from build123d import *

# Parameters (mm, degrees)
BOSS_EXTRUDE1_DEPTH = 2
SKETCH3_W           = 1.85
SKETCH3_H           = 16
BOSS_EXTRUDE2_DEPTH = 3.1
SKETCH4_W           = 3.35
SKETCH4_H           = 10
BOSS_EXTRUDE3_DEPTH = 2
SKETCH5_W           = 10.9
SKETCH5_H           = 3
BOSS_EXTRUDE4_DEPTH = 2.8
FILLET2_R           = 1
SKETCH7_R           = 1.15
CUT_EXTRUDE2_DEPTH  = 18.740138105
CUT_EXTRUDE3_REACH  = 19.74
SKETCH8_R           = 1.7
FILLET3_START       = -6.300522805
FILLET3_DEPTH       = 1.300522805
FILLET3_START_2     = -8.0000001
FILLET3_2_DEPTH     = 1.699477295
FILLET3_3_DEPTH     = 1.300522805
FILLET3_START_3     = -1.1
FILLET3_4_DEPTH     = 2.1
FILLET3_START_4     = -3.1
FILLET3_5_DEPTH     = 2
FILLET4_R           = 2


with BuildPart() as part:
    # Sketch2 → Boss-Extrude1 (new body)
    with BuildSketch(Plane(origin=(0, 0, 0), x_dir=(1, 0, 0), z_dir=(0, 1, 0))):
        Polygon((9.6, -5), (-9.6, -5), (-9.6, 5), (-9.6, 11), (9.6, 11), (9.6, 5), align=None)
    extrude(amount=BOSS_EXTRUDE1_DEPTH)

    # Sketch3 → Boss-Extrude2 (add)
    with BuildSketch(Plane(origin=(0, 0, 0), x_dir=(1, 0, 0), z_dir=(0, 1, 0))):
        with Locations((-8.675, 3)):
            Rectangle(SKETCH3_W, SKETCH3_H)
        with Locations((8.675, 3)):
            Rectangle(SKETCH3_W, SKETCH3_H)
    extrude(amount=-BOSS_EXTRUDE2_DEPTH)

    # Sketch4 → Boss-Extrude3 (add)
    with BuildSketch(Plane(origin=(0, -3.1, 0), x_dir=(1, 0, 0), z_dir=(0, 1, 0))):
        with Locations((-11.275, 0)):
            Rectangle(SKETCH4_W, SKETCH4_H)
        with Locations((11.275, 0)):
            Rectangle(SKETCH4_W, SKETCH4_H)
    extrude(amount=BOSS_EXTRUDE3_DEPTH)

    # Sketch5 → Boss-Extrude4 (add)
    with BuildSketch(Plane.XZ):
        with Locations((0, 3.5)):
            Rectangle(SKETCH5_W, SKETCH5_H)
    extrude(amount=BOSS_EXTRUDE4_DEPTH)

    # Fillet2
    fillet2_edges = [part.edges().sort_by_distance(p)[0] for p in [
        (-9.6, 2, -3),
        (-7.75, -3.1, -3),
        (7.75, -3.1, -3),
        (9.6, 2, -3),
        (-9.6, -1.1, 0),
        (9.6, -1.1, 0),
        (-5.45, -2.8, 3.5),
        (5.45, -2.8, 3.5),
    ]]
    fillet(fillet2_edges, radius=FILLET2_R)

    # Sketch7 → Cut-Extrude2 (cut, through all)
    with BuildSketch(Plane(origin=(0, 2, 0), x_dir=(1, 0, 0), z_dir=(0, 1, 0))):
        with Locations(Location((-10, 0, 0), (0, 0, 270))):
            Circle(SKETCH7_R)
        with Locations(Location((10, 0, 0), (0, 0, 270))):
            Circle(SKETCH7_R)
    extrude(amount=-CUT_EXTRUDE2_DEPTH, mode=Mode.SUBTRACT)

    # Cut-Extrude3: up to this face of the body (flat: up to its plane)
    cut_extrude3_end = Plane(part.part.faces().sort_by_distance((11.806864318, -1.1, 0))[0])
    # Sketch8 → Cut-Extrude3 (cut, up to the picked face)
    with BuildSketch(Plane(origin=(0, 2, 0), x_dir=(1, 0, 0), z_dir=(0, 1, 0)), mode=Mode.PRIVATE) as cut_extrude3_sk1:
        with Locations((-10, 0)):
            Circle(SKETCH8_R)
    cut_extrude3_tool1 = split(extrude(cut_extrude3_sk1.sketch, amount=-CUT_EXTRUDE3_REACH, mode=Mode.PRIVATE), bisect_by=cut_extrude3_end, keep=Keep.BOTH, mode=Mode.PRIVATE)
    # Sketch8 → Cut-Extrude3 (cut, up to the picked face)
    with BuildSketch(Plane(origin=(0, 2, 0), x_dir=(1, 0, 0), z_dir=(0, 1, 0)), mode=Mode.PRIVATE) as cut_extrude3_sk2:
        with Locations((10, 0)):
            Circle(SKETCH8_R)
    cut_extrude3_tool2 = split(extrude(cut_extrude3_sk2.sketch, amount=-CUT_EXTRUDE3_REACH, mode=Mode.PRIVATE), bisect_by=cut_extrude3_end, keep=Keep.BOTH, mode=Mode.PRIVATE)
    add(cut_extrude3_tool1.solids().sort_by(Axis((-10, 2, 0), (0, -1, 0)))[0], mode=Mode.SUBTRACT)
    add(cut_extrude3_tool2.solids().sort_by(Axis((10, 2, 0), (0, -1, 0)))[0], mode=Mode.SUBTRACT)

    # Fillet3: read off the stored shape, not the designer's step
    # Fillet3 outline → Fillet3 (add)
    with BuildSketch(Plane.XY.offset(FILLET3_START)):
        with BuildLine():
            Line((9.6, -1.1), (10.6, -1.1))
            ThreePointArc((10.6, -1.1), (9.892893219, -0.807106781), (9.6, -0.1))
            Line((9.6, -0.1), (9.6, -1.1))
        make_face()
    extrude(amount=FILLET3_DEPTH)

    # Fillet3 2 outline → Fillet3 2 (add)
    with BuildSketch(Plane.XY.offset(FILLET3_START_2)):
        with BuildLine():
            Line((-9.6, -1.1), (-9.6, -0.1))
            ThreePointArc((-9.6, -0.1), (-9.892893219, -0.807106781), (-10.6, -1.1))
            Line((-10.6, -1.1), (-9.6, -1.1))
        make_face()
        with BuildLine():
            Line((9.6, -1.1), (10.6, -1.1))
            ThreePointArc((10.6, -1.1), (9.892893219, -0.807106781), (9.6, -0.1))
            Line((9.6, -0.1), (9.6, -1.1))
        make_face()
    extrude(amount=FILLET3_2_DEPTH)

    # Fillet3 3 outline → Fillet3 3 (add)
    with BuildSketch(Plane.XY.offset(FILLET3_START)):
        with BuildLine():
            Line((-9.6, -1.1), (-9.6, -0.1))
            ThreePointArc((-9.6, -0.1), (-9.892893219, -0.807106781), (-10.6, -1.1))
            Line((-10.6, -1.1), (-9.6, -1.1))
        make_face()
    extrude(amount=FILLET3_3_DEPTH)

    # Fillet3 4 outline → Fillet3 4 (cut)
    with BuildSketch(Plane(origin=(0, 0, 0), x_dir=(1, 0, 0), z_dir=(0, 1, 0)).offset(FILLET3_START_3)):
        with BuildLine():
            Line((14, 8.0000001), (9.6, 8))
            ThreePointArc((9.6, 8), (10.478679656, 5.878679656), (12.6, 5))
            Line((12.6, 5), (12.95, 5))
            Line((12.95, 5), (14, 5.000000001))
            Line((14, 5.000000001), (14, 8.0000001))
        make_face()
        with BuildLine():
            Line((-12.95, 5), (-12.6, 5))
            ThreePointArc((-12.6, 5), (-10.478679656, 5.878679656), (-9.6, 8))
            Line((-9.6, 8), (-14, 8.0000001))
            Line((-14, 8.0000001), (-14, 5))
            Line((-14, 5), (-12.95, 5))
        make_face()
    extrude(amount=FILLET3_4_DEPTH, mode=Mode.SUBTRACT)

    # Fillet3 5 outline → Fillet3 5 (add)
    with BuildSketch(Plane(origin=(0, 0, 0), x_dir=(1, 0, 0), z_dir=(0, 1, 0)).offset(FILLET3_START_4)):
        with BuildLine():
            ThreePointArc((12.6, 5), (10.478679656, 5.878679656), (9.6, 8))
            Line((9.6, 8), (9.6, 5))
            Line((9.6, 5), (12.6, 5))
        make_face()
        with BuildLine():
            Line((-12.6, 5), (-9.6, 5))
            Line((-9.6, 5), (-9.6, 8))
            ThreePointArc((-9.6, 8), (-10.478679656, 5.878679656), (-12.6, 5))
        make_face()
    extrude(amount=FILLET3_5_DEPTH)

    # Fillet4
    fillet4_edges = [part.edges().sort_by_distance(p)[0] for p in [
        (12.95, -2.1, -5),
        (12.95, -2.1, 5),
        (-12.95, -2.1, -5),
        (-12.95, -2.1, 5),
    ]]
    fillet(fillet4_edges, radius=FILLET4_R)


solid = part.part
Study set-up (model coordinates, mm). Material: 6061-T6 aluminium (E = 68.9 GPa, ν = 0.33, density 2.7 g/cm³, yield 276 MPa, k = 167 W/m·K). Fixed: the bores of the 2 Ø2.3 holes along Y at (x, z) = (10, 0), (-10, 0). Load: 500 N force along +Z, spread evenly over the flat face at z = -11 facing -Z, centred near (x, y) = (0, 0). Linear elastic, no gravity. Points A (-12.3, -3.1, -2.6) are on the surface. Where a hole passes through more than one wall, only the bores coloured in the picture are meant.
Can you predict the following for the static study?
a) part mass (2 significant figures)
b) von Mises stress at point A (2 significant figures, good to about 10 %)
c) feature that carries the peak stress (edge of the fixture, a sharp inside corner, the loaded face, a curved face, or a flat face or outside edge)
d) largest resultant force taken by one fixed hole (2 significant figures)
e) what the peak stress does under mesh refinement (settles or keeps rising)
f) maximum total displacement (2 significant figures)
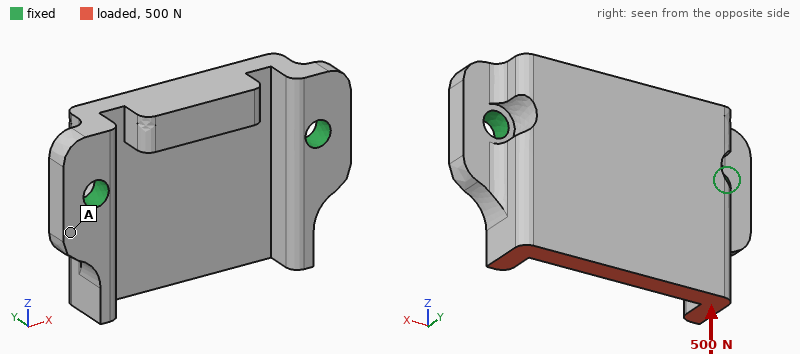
2.6 g
23 MPa
edge of the fixture
250 N
keeps rising
26 µm
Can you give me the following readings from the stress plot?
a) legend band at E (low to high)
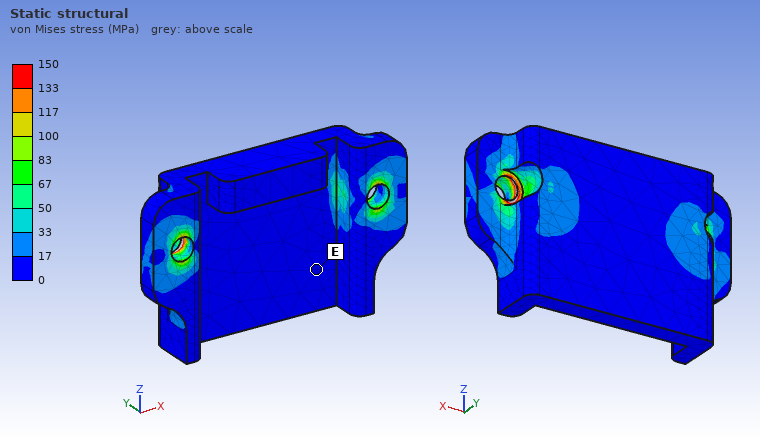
0 to 17 MPa
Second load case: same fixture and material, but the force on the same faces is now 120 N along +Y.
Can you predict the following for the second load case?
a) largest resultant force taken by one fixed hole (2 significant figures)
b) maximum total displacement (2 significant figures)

79 N
38 µm
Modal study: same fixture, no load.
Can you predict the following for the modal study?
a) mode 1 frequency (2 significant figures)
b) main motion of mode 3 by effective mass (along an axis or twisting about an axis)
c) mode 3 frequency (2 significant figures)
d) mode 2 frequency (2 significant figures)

13 kHz
along Y
26 kHz
22 kHz
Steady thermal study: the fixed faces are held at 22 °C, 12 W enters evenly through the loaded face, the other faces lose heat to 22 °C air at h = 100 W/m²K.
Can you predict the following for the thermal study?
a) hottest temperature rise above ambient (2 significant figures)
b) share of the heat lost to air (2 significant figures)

20 K
7.8 %
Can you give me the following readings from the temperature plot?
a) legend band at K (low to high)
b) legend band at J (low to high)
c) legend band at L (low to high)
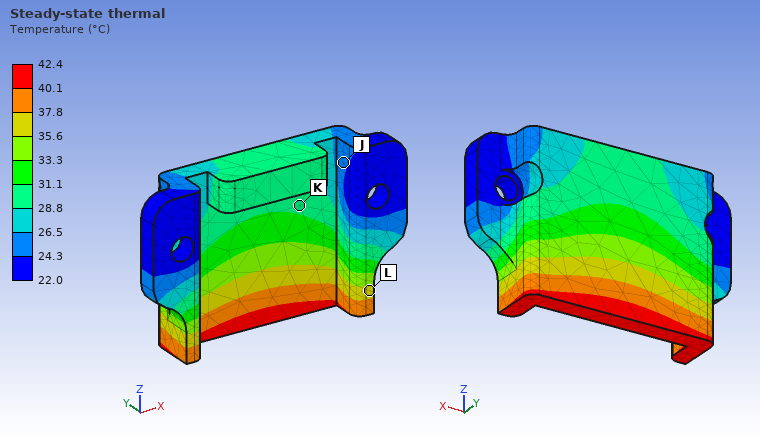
28.8 to 31.1 °C
24.3 to 26.5 °C
35.6 to 37.8 °C
